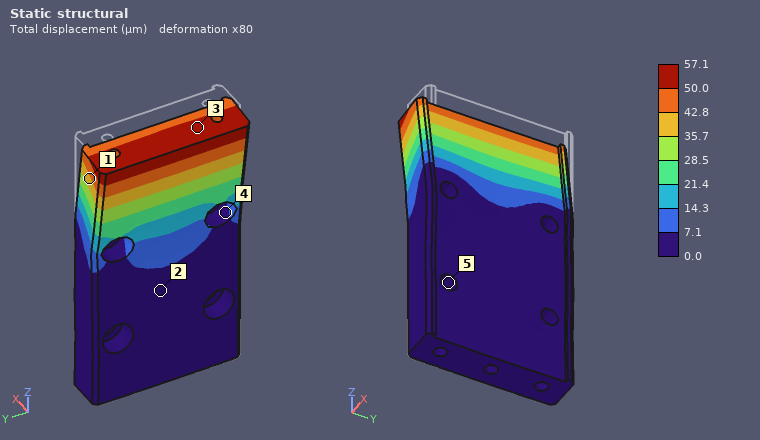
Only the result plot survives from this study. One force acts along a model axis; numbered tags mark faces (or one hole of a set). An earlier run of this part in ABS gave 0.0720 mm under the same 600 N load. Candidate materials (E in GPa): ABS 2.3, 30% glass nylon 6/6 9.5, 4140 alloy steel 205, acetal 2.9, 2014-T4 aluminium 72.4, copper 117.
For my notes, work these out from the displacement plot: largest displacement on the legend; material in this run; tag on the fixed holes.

57.1 µm
acetal
5
